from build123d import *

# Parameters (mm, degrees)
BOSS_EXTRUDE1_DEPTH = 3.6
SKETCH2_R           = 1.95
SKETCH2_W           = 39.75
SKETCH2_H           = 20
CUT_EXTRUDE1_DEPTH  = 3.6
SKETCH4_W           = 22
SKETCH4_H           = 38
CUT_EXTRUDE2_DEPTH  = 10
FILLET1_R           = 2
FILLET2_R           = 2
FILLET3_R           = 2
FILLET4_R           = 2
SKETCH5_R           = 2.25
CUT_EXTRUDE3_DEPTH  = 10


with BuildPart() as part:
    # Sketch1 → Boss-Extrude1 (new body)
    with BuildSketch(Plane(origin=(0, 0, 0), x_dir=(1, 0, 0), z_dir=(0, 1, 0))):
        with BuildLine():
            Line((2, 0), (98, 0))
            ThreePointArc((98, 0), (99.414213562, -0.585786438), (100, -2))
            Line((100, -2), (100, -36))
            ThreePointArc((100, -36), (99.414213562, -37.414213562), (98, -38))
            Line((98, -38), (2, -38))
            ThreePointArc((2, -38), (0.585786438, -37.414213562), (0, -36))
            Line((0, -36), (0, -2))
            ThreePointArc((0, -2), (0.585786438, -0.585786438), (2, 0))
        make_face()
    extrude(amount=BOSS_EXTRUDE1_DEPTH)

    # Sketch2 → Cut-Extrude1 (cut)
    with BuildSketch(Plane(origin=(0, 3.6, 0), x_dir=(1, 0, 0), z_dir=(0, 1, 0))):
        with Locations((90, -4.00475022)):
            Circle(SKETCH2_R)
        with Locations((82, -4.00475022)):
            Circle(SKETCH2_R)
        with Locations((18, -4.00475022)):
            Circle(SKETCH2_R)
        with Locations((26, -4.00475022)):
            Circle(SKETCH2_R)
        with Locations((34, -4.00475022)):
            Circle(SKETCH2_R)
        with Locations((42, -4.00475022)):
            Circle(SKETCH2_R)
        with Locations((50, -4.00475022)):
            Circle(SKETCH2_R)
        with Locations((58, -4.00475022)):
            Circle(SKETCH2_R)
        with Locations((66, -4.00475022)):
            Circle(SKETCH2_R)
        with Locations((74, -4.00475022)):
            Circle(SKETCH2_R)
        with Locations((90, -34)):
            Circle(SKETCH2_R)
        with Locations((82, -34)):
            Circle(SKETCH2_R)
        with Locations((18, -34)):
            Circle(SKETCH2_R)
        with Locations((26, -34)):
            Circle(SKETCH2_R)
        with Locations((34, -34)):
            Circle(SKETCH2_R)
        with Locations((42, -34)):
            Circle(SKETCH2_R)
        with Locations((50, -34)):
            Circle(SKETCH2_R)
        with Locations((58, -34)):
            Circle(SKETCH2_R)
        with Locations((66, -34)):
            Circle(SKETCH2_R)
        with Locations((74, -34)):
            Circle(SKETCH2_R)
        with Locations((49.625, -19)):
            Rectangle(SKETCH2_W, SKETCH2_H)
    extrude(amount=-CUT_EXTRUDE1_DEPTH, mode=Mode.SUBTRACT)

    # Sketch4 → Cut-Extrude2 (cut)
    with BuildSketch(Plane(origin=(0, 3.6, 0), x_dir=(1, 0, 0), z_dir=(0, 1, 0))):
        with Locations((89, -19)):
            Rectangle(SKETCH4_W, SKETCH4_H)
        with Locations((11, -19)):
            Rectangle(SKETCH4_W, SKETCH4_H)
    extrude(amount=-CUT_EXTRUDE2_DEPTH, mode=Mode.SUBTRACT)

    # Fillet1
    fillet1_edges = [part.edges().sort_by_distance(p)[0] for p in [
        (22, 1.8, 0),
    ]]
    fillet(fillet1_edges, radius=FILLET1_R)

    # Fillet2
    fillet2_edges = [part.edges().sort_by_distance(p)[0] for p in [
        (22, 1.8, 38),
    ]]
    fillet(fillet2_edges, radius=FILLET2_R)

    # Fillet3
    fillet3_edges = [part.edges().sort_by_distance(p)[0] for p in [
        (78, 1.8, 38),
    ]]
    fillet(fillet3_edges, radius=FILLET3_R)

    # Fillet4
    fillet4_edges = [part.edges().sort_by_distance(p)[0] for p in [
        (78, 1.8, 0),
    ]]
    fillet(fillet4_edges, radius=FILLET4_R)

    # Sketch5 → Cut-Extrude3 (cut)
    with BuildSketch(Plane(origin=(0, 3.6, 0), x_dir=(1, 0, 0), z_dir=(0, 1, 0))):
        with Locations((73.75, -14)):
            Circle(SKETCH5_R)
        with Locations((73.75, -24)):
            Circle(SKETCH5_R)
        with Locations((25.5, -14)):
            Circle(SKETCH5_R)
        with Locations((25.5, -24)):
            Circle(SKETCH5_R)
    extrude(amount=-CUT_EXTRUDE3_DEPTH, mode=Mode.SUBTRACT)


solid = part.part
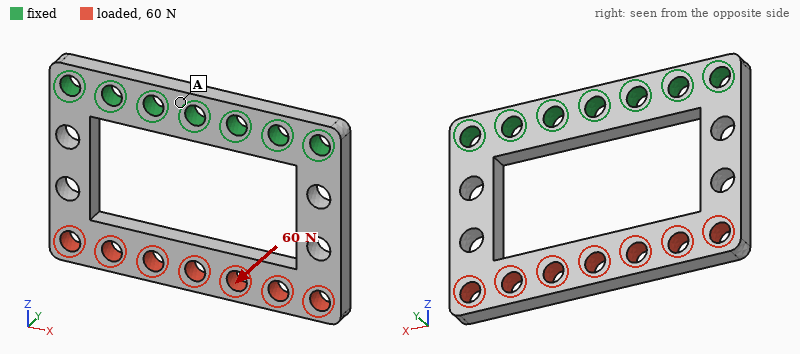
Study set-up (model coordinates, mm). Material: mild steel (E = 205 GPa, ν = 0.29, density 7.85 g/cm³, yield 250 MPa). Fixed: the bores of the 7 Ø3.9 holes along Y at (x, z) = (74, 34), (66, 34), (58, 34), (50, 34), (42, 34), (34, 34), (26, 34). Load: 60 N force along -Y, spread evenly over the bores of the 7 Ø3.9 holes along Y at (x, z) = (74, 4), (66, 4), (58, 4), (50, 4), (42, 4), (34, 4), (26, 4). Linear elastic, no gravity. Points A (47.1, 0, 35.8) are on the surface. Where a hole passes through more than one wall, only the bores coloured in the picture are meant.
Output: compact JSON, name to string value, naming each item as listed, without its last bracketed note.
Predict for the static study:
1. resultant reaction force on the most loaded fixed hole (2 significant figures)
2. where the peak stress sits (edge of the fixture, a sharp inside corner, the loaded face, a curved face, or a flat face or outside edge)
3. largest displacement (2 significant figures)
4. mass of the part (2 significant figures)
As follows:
{"resultant reaction force on the most loaded fixed hole": "24 N", "where the peak stress sits": "a curved face", "largest displacement": "70 µm", "mass of the part": "31 g"}
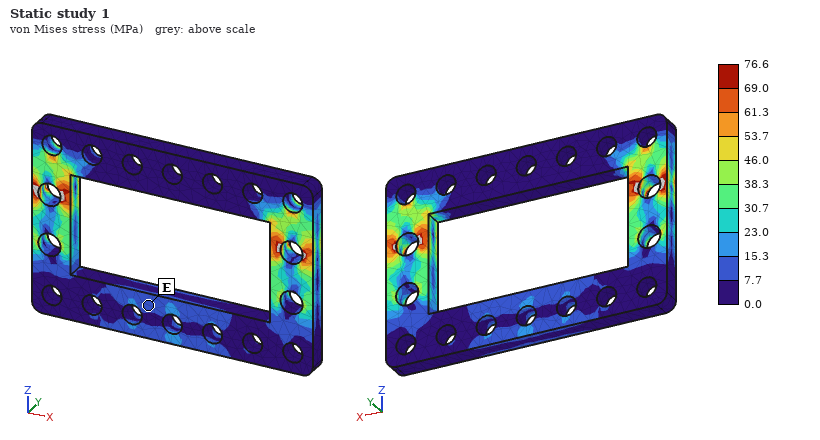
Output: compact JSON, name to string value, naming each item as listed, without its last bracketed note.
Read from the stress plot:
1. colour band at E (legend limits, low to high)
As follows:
{"colour band at E": "7.7 to 15.3 MPa"}
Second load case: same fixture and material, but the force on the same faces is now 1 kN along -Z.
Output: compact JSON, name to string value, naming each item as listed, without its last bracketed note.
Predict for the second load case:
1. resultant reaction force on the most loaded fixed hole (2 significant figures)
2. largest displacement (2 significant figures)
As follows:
{"resultant reaction force on the most loaded fixed hole": "510 N", "largest displacement": "20 µm"}
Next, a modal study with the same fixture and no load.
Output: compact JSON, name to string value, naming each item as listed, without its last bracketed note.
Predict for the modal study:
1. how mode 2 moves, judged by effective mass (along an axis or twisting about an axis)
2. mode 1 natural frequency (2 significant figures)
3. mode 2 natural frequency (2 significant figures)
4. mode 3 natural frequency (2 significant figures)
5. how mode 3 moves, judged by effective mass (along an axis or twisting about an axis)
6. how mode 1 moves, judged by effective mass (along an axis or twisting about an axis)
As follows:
{"how mode 2 moves, judged by effective mass": "twisting about Z", "mode 1 natural frequency": "1500 Hz", "mode 2 natural frequency": "3200 Hz", "mode 3 natural frequency": "5500 Hz", "how mode 3 moves, judged by effective mass": "along X", "how mode 1 moves, judged by effective mass": "along Y"}
